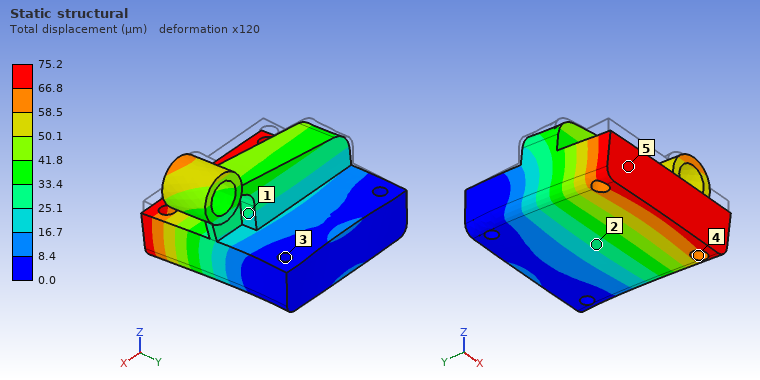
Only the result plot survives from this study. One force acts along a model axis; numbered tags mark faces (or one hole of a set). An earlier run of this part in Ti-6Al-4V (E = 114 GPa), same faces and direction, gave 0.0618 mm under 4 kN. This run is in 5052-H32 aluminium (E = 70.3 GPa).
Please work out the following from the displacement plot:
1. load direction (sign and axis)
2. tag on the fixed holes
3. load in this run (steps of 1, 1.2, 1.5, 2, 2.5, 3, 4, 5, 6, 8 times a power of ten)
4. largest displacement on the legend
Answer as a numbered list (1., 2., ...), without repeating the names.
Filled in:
1. -Z
2. 3
3. 3 kN
4. 75.2 µm
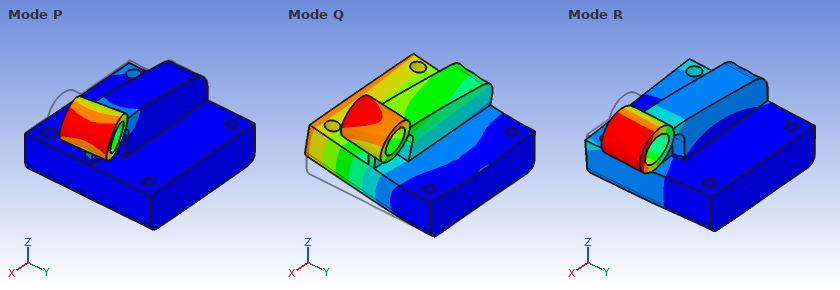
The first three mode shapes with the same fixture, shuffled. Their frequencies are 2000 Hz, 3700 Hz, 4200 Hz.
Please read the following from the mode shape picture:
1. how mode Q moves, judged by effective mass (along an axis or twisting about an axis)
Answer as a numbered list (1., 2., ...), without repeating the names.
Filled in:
1. along Z
